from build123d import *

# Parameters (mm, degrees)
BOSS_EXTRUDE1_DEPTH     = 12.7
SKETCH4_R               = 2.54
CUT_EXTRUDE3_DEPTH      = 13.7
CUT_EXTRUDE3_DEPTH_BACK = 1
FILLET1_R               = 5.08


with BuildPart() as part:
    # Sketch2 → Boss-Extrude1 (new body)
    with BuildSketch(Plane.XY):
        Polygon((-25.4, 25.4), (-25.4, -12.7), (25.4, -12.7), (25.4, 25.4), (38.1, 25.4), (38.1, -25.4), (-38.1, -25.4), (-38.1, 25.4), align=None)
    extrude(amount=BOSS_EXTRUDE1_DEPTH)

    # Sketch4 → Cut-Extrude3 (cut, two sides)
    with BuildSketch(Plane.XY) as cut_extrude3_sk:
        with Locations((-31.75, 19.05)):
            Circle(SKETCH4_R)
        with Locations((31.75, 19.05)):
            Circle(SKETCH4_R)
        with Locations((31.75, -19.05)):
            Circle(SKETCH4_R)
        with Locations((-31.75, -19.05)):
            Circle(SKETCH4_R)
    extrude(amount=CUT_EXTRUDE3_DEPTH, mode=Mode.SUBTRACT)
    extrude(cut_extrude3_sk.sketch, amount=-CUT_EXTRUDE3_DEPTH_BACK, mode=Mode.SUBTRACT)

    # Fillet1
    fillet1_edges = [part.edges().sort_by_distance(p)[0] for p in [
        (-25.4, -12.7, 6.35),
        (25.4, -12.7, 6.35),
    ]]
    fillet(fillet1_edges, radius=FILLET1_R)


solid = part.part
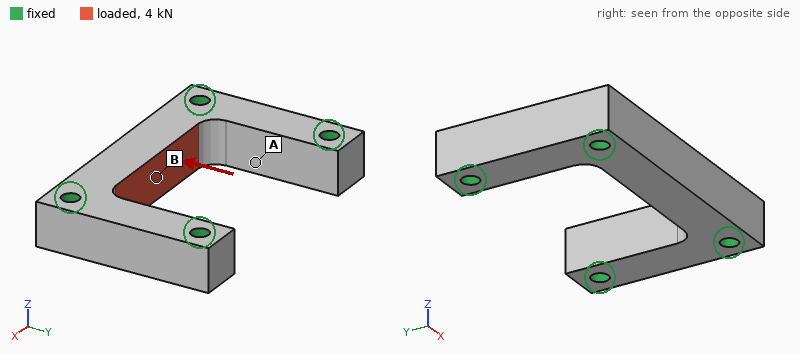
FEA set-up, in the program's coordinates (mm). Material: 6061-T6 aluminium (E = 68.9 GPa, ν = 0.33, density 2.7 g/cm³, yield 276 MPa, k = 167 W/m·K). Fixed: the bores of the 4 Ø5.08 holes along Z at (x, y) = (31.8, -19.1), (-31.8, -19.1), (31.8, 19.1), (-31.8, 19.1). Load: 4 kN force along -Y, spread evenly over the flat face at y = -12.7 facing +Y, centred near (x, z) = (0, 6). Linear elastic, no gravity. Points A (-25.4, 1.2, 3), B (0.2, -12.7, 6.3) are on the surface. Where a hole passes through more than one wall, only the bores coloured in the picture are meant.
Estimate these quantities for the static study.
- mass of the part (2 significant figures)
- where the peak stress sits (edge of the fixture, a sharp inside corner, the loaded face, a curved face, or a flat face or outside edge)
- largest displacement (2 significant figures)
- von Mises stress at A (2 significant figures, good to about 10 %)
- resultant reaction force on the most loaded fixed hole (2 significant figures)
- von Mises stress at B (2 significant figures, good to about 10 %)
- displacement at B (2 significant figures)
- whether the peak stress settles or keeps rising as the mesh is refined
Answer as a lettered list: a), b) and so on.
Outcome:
a) 64 g
b) edge of the fixture
c) 33 µm
d) 13 MPa
e) 1.6 kN
f) 41 MPa
g) 33 µm
h) keeps rising
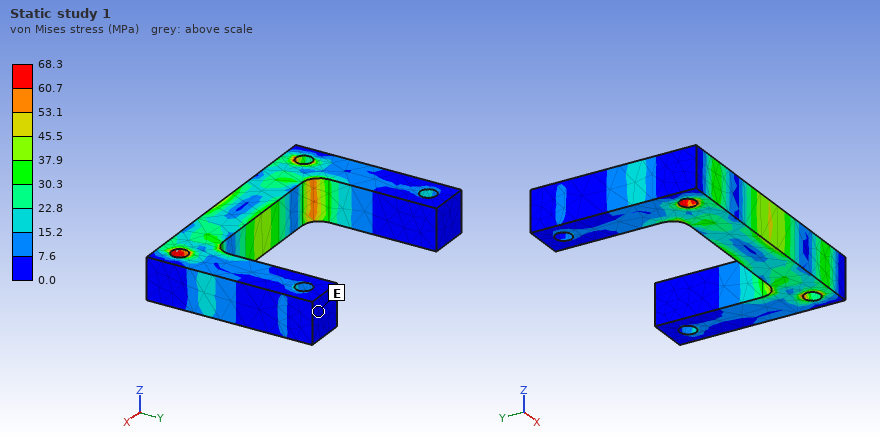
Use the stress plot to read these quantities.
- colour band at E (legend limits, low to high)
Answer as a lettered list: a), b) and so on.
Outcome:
a) 0.0 to 7.6 MPa
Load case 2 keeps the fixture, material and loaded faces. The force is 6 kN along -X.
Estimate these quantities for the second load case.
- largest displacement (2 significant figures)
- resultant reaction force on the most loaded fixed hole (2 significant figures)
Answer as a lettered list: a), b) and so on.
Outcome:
a) 8.6 µm
b) 3.1 kN
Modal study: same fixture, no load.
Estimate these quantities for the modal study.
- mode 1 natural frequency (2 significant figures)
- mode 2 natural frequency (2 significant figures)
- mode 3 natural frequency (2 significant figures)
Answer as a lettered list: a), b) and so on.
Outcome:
a) 14 kHz
b) 14 kHz
c) 25 kHz
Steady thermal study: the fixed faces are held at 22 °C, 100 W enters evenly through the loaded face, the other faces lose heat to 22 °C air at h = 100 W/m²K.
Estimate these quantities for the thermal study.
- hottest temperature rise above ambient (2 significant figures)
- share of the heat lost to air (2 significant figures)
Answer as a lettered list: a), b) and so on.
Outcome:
a) 39 K
b) 5.6 %
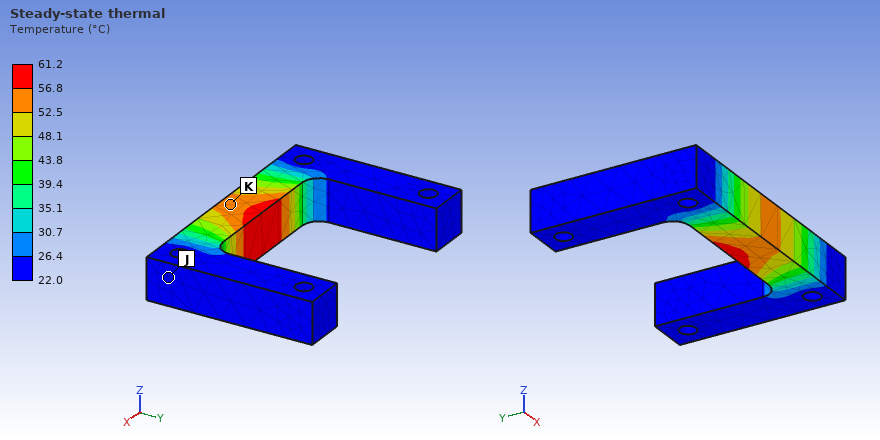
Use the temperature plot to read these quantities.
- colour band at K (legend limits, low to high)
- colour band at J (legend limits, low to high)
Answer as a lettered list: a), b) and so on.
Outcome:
a) 52.5 to 56.8 °C
b) 22.0 to 26.4 °C
